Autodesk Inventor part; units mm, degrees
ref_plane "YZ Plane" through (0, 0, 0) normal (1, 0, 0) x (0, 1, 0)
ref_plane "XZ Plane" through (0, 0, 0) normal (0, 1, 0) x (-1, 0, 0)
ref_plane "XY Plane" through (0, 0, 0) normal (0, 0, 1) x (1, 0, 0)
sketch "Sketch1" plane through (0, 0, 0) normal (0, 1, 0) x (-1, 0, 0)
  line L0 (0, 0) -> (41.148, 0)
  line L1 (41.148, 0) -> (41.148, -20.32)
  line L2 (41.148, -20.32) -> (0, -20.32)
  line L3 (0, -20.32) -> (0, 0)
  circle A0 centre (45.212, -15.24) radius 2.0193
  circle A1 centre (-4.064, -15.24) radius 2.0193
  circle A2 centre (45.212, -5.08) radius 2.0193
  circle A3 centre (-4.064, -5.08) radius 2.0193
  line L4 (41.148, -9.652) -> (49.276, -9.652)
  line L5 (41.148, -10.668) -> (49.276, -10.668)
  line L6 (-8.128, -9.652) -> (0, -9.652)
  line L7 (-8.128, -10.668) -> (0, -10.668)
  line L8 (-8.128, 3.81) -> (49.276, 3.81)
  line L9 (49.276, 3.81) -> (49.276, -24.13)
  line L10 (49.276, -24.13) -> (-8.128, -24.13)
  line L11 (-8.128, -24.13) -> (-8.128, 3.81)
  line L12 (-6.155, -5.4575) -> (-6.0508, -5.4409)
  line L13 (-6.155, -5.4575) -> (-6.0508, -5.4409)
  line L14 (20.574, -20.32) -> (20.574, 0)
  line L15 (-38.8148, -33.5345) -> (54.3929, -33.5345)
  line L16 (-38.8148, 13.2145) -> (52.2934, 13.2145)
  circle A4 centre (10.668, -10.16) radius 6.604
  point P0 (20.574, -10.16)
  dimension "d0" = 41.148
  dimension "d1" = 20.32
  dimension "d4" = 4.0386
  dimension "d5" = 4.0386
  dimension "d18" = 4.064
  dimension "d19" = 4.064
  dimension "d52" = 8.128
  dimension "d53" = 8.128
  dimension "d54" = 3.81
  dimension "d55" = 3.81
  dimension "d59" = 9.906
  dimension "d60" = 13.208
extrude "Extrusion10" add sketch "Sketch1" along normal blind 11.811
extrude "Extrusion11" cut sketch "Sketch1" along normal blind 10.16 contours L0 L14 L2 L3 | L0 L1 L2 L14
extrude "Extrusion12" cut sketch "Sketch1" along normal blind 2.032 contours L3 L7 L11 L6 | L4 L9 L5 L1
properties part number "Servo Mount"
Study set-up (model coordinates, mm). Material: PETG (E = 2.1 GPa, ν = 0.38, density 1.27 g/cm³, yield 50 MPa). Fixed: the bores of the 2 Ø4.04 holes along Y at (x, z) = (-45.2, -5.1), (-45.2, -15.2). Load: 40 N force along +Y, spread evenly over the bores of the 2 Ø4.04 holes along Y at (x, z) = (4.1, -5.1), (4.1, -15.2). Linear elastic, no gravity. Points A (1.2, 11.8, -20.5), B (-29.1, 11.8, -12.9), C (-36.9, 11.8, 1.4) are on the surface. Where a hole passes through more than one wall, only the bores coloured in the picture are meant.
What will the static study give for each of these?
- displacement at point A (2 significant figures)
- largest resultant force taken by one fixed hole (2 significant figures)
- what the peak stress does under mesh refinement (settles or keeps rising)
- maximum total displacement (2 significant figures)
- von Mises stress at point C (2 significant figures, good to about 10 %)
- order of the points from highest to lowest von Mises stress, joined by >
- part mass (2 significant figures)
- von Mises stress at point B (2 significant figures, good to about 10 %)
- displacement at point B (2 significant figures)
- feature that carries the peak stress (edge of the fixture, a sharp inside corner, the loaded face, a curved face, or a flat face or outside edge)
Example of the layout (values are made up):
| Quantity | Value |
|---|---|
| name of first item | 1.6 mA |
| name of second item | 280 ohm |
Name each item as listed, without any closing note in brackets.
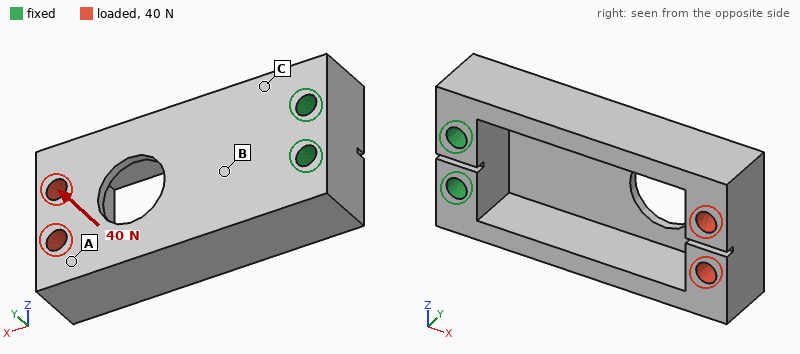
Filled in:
| Quantity | Value |
|---|---|
| displacement at point A | 0.57 mm |
| largest resultant force taken by one fixed hole | 23 N |
| what the peak stress does under mesh refinement | keeps rising |
| maximum total displacement | 0.71 mm |
| von Mises stress at point C | 4.3 MPa |
| order of the points from highest to lowest von Mises stress, joined by > | C > B > A |
| part mass | 12 g |
| von Mises stress at point B | 2.9 MPa |
| displacement at point B | 0.12 mm |
| feature that carries the peak stress | edge of the fixture |
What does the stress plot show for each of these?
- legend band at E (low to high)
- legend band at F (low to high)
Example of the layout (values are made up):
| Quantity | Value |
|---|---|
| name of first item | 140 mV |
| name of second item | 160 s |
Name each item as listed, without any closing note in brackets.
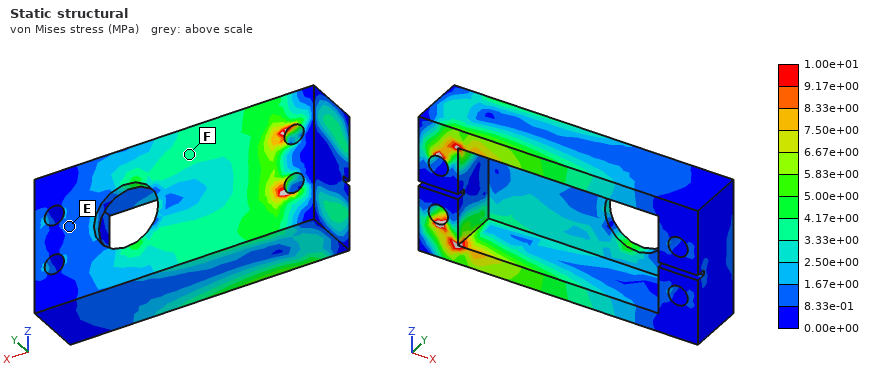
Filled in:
| Quantity | Value |
|---|---|
| legend band at E | 8.33e-01 to 1.67e+00 MPa |
| legend band at F | 3.33e+00 to 4.17e+00 MPa |
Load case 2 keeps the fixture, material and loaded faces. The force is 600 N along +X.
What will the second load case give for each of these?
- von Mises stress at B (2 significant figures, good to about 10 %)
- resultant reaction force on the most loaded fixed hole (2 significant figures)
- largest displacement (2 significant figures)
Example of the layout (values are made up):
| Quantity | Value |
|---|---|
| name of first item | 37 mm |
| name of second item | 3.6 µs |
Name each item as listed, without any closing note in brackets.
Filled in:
| Quantity | Value |
|---|---|
| von Mises stress at B | 3.1 MPa |
| resultant reaction force on the most loaded fixed hole | 300 N |
| largest displacement | 0.60 mm |
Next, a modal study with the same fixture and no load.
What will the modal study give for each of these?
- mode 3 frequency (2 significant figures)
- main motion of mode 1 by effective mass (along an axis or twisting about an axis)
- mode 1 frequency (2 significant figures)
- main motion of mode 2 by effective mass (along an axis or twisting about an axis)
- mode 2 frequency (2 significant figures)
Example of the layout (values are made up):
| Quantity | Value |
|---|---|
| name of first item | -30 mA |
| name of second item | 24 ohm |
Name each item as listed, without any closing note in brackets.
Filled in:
| Quantity | Value |
|---|---|
| mode 3 frequency | 1600 Hz |
| main motion of mode 1 by effective mass | along Y |
| mode 1 frequency | 610 Hz |
| main motion of mode 2 by effective mass | along Z |
| mode 2 frequency | 760 Hz |
